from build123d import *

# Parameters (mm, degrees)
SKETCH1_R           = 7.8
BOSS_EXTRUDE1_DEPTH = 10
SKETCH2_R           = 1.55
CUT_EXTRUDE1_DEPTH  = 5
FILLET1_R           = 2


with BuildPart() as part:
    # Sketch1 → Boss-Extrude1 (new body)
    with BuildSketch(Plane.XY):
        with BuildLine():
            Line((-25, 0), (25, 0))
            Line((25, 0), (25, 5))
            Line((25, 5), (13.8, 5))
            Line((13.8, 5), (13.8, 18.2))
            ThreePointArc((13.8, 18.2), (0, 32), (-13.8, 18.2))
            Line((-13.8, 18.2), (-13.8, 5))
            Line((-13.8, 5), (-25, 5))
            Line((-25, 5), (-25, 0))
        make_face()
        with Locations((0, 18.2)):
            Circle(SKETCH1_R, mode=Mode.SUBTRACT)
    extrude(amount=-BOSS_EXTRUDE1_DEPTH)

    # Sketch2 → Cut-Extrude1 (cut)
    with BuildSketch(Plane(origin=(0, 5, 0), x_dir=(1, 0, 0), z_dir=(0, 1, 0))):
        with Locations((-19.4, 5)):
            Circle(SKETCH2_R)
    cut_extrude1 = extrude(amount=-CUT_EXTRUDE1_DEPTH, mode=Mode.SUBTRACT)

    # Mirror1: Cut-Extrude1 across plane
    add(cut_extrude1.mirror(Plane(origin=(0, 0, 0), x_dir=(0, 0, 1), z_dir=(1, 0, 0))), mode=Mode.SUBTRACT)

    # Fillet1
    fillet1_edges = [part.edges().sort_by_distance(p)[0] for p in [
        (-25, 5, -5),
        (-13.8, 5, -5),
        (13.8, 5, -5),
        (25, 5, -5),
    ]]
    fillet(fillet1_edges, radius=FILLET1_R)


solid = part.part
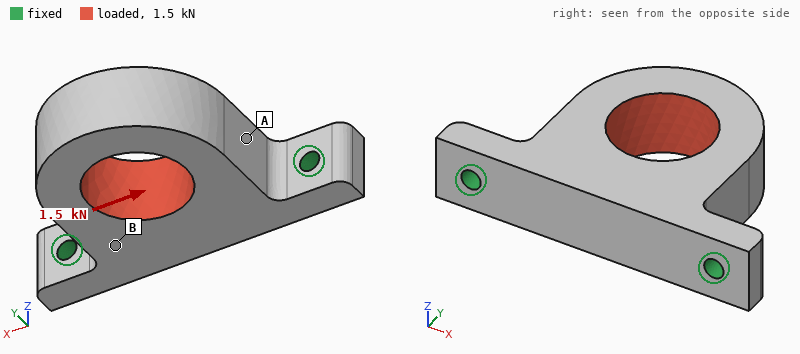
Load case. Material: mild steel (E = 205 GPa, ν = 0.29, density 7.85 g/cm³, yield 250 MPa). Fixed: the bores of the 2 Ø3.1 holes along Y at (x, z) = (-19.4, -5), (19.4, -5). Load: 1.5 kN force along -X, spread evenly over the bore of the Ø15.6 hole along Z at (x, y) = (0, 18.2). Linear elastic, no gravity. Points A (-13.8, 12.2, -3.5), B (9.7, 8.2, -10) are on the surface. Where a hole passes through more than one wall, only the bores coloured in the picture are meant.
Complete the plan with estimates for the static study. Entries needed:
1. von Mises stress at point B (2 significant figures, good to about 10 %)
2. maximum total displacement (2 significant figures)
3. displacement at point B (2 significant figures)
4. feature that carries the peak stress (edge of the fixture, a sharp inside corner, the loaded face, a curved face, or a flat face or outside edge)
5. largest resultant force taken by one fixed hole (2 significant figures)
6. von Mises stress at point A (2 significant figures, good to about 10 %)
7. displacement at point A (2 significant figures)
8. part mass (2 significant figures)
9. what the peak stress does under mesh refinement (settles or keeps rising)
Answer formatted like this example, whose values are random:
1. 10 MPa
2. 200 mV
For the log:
1. 9.2 MPa
2. 9.6 µm
3. 1.7 µm
4. edge of the fixture
5. 1.0 kN
6. 26 MPa
7. 3.8 µm
8. 56 g
9. keeps rising
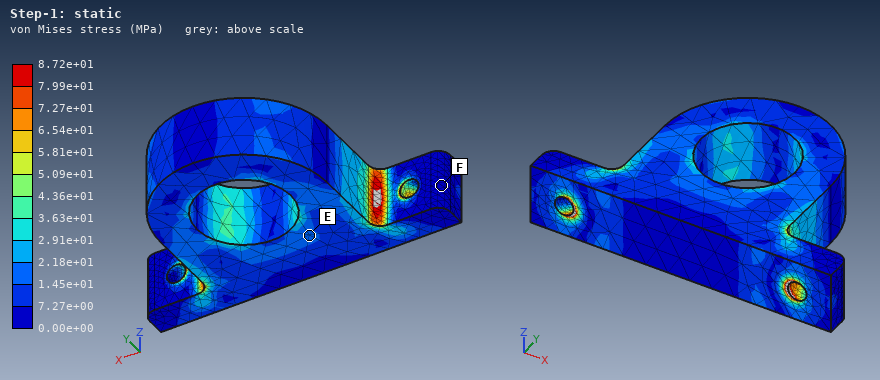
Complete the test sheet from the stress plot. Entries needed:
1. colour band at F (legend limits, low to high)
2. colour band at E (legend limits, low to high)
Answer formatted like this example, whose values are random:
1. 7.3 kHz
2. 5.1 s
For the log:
1. 0.00e+00 to 7.27e+00 MPa
2. 1.45e+01 to 2.18e+01 MPa
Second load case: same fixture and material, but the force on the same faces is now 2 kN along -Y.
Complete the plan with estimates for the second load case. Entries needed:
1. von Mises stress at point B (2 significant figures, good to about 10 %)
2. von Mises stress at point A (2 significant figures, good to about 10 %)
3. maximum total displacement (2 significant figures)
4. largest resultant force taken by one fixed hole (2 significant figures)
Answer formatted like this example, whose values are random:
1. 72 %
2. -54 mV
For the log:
1. 15 MPa
2. 19 MPa
3. 5.0 µm
4. 1.1 kN
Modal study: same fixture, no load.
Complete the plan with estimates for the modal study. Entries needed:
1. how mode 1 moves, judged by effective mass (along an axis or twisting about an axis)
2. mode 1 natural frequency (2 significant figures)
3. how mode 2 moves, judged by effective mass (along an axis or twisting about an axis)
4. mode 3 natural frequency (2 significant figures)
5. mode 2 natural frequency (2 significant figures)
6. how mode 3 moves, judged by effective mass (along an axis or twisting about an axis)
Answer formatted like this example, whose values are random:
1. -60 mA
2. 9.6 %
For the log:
1. along Z
2. 4000 Hz
3. along X
4. 15 kHz
5. 12 kHz
6. along Y
